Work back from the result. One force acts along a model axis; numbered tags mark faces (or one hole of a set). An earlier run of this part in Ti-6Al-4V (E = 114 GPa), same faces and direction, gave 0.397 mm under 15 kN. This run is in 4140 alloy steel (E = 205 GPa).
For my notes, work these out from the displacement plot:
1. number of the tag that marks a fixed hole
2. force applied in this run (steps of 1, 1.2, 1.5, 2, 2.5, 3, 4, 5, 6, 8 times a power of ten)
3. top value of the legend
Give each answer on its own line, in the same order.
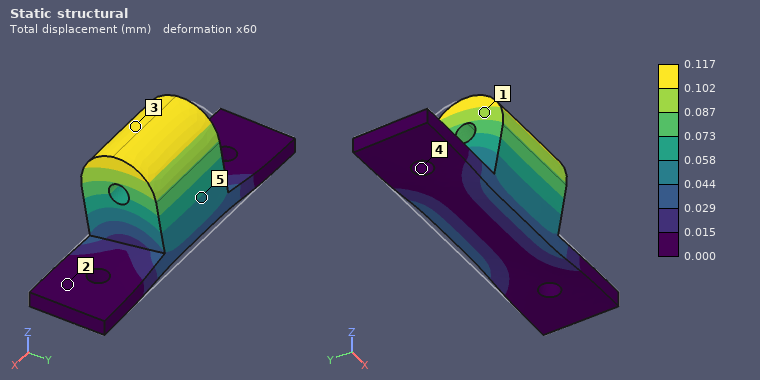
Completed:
4
8 kN
0.117 mm
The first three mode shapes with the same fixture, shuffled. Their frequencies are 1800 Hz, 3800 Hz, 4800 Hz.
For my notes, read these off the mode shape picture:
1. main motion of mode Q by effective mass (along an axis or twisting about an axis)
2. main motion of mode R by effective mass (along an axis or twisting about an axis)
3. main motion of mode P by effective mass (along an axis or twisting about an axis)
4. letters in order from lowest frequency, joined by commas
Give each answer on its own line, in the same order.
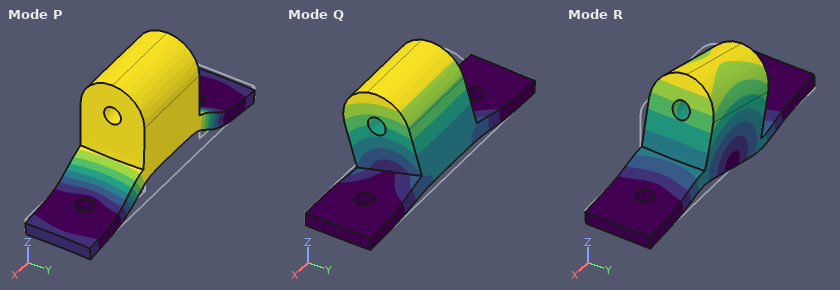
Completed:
along Y
along X
along Z
Q, P, R
